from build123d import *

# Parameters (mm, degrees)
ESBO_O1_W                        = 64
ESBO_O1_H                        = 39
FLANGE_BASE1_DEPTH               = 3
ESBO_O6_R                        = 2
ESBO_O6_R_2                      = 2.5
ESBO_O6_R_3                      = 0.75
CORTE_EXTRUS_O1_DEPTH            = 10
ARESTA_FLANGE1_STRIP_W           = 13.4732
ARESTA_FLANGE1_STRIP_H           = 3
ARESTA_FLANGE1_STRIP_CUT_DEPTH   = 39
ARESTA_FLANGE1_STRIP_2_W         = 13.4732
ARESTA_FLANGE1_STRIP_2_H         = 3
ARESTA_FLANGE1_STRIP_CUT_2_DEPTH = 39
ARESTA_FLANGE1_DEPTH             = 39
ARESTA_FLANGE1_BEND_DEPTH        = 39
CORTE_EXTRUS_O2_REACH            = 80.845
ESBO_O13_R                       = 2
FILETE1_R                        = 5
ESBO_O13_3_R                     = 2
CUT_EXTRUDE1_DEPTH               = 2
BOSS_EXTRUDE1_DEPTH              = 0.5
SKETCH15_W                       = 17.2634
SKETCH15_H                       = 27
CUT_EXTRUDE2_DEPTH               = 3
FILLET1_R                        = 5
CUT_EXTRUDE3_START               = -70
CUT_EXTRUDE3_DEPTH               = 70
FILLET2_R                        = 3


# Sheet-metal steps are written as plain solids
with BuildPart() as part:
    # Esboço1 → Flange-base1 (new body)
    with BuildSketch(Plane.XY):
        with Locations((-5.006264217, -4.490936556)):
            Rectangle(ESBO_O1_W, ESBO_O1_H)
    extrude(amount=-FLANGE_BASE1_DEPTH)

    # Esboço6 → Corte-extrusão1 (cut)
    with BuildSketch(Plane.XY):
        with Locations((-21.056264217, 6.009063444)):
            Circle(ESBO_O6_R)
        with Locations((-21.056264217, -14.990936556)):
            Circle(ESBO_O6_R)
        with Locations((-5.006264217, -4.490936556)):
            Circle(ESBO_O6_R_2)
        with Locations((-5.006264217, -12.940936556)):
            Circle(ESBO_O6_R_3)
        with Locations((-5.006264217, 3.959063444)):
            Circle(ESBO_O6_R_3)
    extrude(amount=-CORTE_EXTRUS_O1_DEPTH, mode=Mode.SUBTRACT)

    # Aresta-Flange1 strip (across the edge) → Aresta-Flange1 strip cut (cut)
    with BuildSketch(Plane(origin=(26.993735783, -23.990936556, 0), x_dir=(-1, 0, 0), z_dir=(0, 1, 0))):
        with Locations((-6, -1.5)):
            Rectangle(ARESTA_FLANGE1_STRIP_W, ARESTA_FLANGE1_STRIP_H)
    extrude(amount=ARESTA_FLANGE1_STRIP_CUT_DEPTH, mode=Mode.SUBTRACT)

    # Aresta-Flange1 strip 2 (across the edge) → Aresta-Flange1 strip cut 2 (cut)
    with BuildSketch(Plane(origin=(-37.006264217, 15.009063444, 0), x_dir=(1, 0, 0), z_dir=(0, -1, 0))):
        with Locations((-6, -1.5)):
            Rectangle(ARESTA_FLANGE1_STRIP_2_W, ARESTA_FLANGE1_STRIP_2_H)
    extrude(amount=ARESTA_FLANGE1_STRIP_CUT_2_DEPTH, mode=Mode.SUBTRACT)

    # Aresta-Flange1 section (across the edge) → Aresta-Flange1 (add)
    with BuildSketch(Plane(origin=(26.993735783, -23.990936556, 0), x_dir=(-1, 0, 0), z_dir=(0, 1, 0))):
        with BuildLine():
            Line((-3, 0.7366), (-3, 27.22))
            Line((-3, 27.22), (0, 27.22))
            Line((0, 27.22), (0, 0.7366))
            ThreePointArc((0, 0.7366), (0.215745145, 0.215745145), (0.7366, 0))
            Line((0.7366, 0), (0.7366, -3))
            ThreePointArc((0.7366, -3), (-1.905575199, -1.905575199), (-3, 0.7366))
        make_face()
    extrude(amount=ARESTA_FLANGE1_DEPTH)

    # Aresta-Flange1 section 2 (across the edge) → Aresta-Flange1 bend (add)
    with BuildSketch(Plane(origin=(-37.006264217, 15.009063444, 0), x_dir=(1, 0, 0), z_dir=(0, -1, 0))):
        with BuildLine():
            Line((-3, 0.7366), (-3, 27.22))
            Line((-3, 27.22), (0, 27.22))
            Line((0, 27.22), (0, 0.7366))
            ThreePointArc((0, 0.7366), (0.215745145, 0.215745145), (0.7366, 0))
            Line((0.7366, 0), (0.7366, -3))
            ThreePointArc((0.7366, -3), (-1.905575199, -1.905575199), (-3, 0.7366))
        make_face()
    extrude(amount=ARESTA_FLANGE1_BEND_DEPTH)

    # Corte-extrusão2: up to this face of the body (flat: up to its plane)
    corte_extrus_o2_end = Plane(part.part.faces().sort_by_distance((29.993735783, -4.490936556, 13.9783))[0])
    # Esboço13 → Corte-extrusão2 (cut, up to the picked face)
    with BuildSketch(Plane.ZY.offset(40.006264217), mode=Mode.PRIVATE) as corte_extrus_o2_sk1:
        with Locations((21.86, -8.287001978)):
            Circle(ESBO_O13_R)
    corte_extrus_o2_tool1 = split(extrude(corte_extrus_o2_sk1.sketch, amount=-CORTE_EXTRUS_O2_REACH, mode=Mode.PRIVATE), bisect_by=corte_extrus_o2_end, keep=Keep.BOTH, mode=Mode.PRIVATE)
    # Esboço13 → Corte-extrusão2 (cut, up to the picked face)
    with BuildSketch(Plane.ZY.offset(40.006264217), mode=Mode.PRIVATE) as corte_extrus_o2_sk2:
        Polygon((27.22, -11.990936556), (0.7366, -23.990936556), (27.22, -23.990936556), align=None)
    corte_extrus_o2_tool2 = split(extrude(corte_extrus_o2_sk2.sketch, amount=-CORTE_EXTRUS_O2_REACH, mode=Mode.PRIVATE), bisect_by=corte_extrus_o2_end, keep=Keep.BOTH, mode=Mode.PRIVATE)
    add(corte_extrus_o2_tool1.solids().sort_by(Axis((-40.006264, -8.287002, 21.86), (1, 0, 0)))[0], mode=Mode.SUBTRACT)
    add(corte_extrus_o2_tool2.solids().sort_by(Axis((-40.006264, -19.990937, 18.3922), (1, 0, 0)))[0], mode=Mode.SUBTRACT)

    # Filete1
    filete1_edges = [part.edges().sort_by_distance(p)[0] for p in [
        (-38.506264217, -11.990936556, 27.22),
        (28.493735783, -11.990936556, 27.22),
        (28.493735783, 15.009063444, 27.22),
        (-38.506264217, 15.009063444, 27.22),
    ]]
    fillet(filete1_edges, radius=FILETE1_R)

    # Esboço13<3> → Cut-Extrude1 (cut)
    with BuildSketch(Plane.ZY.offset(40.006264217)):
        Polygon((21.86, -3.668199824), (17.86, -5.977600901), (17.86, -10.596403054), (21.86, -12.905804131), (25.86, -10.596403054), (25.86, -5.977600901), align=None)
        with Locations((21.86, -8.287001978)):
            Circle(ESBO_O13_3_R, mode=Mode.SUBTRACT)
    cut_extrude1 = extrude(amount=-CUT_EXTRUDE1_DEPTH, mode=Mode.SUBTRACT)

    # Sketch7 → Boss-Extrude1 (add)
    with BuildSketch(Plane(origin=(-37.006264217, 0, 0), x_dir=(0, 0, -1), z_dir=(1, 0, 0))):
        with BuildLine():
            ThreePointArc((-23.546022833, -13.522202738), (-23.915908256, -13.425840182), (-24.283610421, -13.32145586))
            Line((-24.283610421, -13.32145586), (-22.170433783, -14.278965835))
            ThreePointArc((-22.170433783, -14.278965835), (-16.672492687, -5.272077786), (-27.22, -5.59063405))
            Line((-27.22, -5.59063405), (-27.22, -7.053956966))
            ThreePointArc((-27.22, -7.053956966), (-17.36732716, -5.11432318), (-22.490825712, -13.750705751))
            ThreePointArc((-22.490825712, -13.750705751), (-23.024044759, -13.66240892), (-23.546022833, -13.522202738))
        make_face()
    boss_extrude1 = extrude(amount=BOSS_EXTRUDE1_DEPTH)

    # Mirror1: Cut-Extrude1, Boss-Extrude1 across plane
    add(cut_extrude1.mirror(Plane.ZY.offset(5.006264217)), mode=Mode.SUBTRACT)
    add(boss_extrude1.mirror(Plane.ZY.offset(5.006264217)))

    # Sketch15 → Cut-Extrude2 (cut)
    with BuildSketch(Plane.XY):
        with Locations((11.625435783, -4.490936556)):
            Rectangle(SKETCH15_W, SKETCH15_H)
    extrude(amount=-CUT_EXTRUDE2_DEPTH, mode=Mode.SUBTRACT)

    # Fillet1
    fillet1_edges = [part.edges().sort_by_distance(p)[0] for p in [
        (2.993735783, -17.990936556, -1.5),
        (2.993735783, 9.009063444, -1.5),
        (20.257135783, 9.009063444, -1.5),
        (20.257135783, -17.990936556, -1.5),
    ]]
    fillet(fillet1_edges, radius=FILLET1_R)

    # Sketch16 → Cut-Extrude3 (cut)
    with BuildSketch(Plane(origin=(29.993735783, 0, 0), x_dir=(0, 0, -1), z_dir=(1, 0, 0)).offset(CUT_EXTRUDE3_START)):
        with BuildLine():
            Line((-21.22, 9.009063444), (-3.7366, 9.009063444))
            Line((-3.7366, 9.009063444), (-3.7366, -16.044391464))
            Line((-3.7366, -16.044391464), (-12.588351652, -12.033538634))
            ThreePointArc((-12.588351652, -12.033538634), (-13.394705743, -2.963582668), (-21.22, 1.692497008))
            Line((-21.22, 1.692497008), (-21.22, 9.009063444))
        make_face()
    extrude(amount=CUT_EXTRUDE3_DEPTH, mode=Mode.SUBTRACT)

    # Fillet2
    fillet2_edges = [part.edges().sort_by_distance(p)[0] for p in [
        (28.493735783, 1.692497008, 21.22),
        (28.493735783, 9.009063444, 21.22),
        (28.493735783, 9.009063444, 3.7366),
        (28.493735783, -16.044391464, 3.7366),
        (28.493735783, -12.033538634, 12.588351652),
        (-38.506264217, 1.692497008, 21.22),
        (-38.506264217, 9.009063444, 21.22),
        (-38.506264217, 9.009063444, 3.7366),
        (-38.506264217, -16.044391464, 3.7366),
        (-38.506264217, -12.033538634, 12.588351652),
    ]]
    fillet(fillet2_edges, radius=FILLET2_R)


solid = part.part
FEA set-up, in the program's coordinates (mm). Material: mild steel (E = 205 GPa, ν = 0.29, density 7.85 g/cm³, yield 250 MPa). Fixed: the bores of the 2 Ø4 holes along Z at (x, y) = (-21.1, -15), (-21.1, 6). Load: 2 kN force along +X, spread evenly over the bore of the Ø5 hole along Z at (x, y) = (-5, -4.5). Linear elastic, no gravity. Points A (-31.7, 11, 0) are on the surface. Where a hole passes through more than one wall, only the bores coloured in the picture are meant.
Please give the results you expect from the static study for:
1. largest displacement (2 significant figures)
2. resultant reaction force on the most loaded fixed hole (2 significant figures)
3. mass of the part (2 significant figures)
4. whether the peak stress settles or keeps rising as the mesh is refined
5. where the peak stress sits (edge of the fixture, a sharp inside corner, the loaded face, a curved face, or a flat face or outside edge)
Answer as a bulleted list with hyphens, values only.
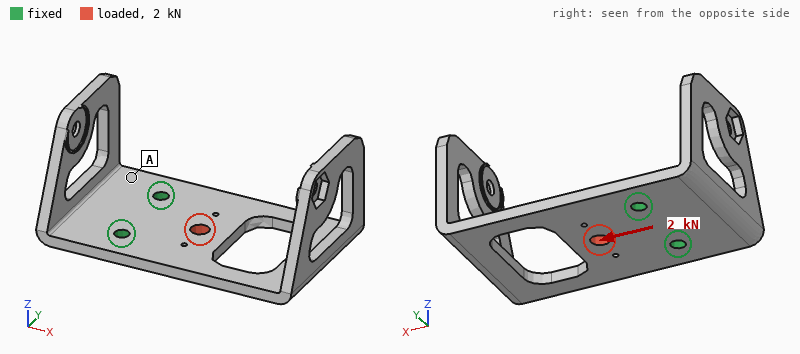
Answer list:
- 4.1 µm
- 1.0 kN
- 79 g
- keeps rising
- a sharp inside corner
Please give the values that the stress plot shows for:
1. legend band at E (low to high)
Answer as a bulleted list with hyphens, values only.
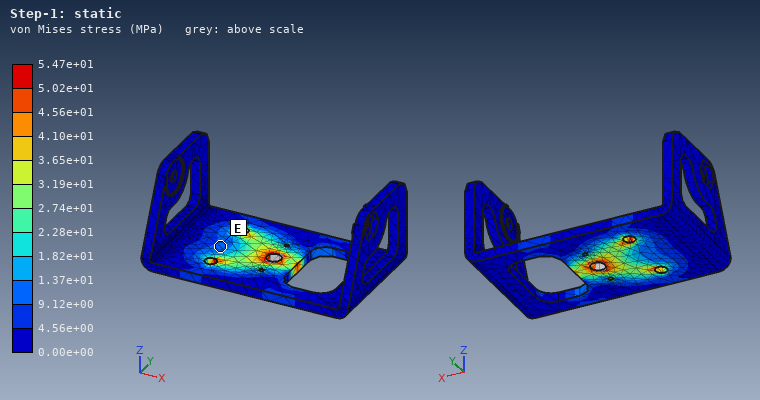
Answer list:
- 9.12e+00 to 1.37e+01 MPa
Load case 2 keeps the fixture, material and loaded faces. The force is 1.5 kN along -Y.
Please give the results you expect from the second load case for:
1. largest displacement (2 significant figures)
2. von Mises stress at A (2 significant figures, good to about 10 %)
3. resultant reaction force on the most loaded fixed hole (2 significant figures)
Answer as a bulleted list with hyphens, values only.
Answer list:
- 10 µm
- 4.7 MPa
- 1.2 kN
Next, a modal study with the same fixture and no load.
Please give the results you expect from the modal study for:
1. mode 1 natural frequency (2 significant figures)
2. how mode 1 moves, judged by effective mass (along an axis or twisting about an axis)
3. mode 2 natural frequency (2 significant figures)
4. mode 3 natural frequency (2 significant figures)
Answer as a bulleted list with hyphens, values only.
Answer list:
- 550 Hz
- along Z
- 1300 Hz
- 1700 Hz
